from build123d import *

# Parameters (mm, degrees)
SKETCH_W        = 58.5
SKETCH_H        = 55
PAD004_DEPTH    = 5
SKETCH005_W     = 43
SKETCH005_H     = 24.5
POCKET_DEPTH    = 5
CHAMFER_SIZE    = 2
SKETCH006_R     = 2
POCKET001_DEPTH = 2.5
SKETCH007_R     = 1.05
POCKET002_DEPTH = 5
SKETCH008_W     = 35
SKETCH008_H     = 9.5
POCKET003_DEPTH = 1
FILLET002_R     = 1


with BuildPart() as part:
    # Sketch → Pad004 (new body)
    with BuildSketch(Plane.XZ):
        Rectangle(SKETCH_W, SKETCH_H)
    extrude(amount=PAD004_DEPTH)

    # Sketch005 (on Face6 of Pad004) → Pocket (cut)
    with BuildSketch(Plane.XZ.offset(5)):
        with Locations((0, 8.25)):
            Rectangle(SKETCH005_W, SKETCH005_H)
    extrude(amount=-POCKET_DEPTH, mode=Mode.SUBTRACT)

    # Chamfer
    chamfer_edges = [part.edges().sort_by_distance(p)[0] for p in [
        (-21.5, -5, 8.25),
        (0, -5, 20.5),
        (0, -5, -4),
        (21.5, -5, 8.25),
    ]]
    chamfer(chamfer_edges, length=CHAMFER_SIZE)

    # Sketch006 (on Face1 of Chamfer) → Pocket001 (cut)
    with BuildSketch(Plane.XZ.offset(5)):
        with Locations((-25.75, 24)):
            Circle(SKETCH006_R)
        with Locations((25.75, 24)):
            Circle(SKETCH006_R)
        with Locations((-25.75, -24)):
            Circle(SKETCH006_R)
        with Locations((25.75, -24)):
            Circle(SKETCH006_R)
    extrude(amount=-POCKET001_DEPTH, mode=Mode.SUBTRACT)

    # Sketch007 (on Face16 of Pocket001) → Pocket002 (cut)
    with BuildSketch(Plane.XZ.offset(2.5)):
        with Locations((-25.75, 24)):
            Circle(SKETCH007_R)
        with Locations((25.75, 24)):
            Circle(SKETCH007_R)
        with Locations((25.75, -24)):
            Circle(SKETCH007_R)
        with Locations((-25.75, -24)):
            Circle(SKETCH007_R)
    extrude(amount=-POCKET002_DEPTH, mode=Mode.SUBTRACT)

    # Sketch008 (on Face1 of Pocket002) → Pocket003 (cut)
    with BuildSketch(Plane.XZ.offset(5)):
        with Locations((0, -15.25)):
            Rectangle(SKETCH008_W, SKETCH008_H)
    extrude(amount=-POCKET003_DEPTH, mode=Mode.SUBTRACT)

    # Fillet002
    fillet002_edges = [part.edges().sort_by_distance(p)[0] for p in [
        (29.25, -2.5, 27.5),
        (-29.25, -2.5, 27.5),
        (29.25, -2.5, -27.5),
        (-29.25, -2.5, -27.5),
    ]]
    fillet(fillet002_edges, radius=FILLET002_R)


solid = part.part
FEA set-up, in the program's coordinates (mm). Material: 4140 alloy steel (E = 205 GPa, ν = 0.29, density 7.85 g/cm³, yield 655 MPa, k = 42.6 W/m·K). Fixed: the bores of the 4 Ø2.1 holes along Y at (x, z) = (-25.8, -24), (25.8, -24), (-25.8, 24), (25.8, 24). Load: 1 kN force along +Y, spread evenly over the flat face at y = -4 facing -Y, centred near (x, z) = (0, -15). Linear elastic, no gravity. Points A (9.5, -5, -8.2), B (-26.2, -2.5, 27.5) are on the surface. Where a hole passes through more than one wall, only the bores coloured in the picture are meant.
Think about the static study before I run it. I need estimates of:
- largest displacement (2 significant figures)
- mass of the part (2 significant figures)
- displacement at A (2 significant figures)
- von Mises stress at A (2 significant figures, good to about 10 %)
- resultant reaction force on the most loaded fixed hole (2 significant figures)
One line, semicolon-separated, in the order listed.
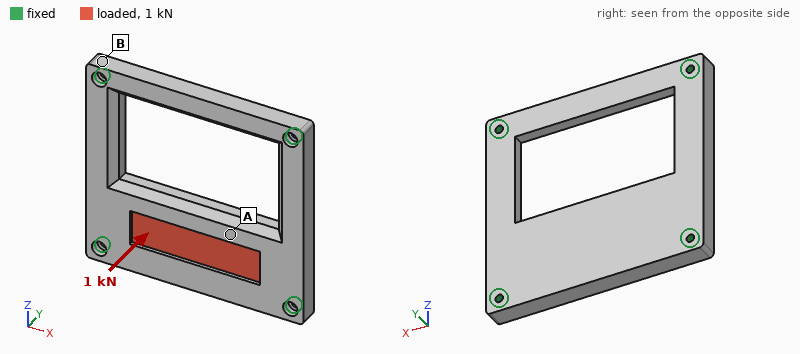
44 µm; 79 g; 35 µm; 52 MPa; 600 N
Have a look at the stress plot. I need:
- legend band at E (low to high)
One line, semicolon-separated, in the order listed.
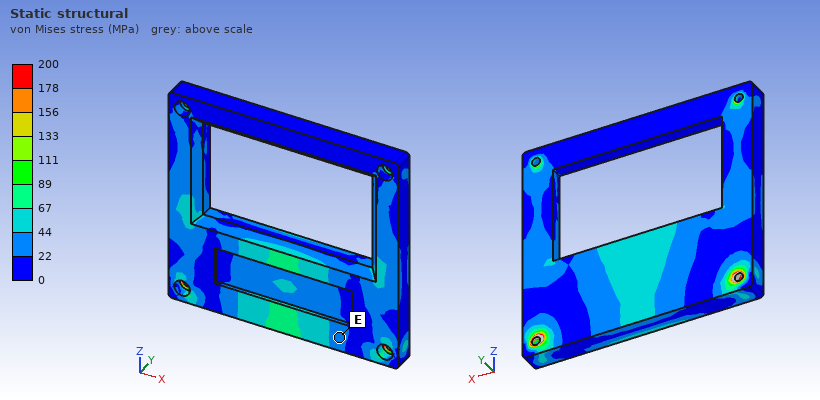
22 to 44 MPa
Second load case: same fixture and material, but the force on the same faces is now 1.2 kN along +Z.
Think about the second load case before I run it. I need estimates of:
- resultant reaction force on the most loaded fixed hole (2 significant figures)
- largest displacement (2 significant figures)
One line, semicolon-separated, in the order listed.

540 N; 8.7 µm
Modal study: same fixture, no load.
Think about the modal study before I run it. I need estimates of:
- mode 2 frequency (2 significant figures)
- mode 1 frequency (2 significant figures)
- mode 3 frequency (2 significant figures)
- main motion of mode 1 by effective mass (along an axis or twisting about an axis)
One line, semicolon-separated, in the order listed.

7600 Hz; 4900 Hz; 8400 Hz; along Y
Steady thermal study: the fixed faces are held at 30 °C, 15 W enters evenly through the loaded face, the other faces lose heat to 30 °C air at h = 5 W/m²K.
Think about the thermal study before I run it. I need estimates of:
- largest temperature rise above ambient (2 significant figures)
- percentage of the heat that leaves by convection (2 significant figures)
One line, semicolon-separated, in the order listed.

46 K; 3.7 %
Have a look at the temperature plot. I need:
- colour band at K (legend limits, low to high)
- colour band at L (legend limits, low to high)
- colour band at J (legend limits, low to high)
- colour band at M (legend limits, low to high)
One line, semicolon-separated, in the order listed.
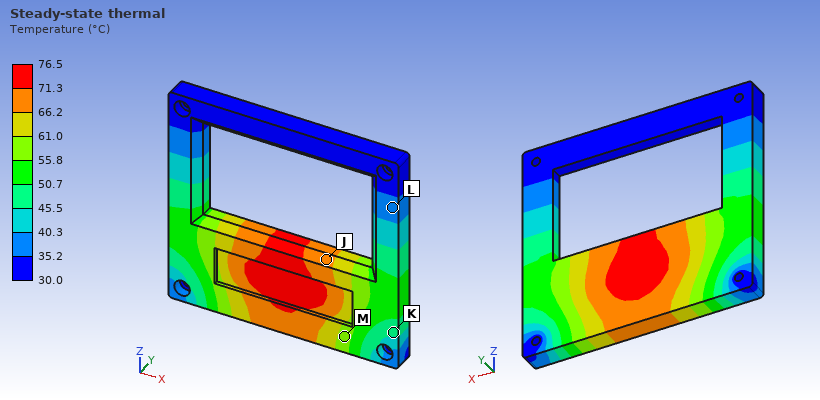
45.5 to 50.7 °C; 35.2 to 40.3 °C; 66.2 to 71.3 °C; 55.8 to 61.0 °C
